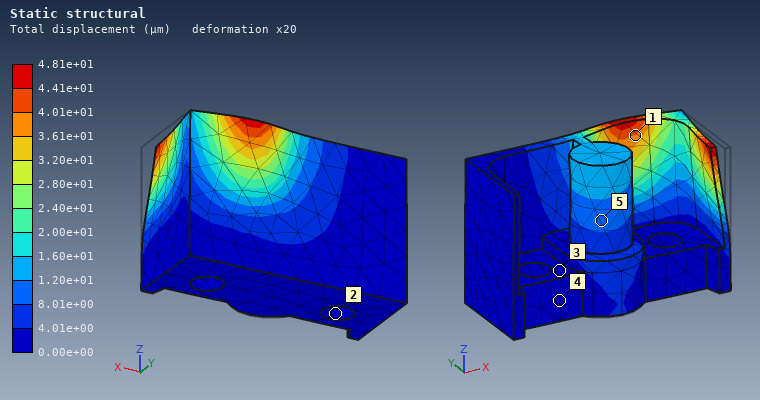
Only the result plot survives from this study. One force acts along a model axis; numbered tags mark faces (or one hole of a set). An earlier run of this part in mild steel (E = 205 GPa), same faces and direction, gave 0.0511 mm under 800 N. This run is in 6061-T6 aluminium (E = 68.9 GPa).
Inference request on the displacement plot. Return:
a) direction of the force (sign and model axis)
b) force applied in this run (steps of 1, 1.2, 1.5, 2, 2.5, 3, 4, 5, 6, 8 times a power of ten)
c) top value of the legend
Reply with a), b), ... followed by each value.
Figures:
a) +Y
b) 250 N
c) 4.81e+01 µm
